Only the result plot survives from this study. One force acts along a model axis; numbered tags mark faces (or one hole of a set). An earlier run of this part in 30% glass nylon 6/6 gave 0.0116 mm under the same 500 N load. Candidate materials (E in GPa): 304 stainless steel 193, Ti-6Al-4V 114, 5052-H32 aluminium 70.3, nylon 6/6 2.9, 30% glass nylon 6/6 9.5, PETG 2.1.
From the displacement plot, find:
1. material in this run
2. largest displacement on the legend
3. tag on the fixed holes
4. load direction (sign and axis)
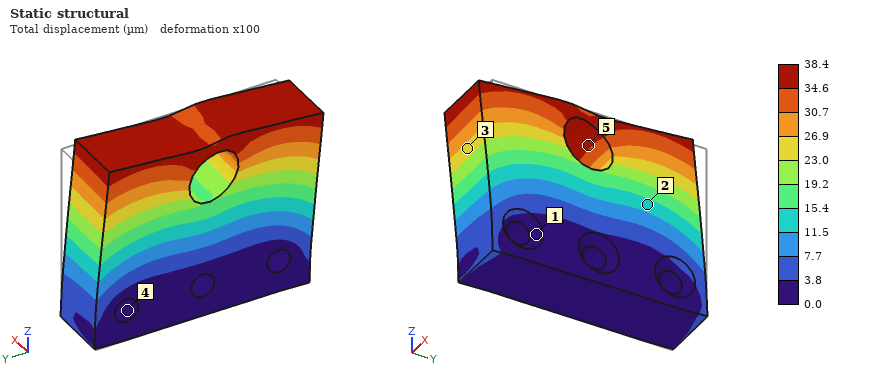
nylon 6/6
38.4 µm
4
-Y
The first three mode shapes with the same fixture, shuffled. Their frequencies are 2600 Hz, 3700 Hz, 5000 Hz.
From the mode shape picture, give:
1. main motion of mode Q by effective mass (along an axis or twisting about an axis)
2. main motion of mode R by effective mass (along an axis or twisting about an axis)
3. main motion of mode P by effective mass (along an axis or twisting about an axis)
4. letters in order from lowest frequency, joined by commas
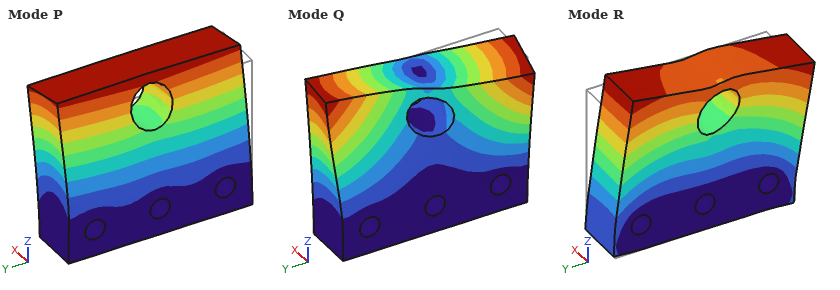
twisting about Z
along Y
along X
P, Q, R
